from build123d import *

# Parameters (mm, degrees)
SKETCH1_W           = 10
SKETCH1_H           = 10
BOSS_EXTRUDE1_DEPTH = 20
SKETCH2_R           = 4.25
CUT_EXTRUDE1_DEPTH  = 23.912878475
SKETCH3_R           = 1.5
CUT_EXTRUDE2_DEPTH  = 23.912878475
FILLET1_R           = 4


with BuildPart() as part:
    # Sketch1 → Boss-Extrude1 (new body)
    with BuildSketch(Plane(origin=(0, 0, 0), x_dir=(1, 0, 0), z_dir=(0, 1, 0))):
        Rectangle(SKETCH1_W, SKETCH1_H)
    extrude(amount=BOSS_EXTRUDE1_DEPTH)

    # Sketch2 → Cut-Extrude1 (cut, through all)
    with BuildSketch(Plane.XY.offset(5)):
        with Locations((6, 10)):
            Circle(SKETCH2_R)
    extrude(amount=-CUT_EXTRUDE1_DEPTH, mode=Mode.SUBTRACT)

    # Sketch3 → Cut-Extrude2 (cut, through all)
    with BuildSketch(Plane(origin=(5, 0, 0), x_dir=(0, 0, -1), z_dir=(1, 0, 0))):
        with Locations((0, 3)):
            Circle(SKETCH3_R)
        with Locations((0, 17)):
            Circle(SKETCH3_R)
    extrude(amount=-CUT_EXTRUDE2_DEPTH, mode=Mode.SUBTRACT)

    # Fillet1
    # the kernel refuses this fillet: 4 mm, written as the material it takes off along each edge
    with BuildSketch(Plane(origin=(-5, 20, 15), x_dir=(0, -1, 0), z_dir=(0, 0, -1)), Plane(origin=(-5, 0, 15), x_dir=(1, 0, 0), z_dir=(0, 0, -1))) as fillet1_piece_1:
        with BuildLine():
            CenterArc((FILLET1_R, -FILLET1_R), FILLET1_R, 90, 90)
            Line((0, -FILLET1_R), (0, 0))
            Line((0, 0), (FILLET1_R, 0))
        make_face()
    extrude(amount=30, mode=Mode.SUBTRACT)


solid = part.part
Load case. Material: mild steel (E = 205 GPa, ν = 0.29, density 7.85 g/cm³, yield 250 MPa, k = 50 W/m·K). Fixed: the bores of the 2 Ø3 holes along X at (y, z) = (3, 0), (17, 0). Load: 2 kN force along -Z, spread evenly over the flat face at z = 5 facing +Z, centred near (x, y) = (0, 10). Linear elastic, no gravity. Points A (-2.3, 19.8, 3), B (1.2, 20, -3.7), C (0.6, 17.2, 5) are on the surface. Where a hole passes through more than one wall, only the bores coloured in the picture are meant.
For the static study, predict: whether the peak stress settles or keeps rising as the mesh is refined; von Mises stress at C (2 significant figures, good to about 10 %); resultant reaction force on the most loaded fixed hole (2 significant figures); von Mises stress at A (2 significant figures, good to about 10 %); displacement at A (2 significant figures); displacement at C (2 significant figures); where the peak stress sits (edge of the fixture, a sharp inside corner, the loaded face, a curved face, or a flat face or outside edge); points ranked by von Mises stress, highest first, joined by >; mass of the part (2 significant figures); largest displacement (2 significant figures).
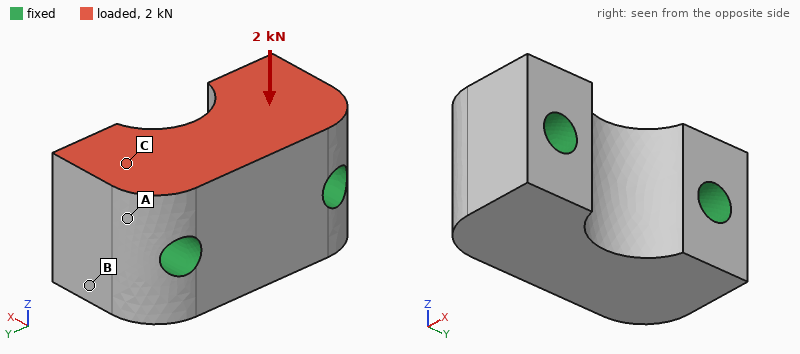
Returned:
keeps rising
15 MPa
1.0 kN
7.9 MPa
0.12 µm
0.24 µm
edge of the fixture
C > A > B
13 g
0.69 µm
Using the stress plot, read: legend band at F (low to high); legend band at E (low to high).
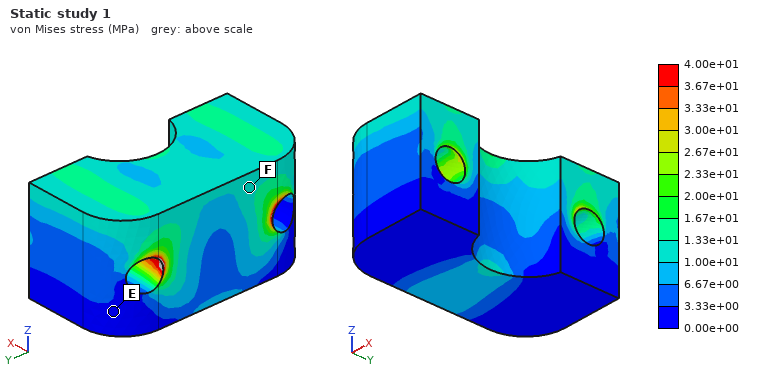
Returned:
1.00e+01 to 1.33e+01 MPa
0.00e+00 to 3.33e+00 MPa
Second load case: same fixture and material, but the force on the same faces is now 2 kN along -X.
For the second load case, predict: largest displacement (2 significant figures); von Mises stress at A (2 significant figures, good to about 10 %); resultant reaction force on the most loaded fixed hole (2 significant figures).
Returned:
2.0 µm
17 MPa
1.0 kN
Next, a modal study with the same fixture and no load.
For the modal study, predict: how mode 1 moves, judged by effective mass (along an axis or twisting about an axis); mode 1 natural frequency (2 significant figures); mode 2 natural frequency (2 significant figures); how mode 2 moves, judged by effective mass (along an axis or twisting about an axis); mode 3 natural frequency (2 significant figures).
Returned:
along Z
96 kHz
110 kHz
along X
120 kHz
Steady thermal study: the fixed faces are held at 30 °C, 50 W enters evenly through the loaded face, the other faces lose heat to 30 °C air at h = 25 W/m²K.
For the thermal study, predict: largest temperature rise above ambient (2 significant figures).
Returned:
34 K
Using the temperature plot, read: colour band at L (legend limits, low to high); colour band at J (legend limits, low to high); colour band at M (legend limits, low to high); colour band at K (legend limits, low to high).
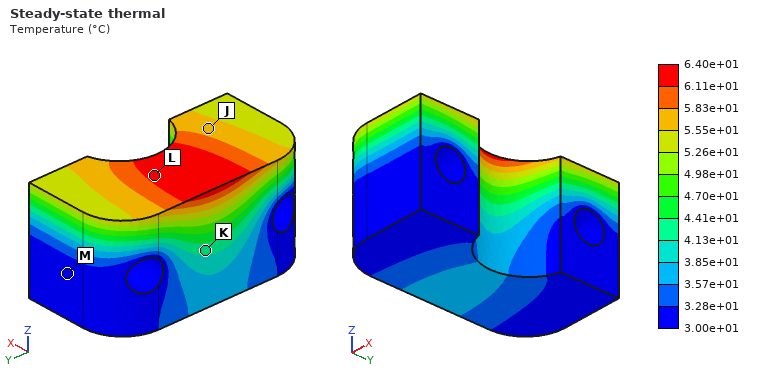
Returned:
6.11e+01 to 6.40e+01 °C
5.55e+01 to 5.83e+01 °C
3.00e+01 to 3.28e+01 °C
4.13e+01 to 4.41e+01 °C
